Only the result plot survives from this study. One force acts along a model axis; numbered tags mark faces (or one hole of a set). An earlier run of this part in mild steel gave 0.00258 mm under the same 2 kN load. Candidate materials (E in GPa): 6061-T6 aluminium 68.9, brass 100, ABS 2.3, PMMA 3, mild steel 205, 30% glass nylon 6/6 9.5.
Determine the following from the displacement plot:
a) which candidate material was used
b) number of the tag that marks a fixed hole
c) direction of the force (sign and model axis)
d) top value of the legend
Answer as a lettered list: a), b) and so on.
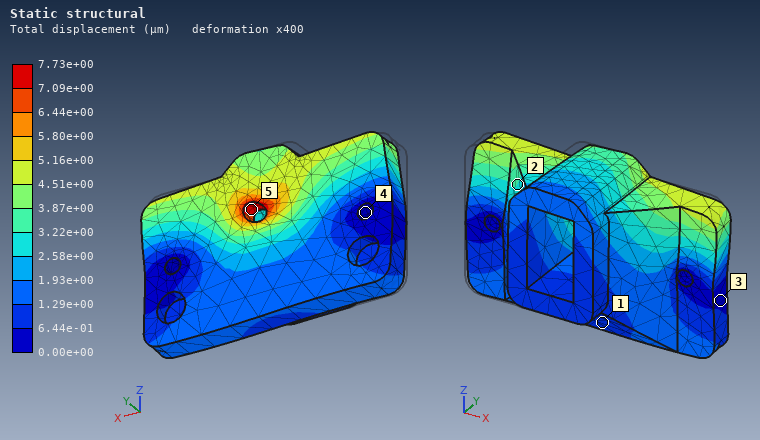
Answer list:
a) 6061-T6 aluminium
b) 4
c) +X
d) 7.73e+00 µm
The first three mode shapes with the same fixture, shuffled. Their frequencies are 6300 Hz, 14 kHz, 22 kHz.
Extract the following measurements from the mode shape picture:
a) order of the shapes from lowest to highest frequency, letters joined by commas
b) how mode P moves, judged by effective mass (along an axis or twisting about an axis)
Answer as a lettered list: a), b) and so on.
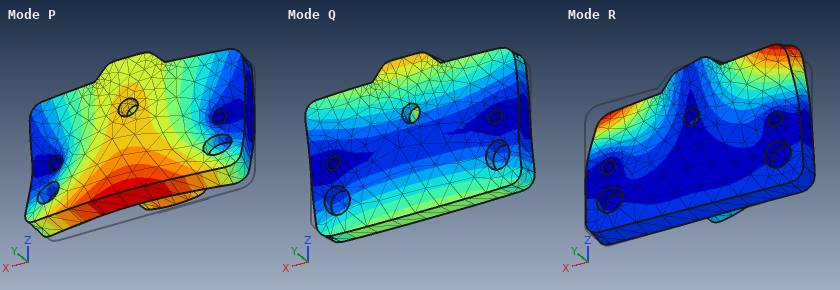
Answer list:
a) Q, P, R
b) along Y
